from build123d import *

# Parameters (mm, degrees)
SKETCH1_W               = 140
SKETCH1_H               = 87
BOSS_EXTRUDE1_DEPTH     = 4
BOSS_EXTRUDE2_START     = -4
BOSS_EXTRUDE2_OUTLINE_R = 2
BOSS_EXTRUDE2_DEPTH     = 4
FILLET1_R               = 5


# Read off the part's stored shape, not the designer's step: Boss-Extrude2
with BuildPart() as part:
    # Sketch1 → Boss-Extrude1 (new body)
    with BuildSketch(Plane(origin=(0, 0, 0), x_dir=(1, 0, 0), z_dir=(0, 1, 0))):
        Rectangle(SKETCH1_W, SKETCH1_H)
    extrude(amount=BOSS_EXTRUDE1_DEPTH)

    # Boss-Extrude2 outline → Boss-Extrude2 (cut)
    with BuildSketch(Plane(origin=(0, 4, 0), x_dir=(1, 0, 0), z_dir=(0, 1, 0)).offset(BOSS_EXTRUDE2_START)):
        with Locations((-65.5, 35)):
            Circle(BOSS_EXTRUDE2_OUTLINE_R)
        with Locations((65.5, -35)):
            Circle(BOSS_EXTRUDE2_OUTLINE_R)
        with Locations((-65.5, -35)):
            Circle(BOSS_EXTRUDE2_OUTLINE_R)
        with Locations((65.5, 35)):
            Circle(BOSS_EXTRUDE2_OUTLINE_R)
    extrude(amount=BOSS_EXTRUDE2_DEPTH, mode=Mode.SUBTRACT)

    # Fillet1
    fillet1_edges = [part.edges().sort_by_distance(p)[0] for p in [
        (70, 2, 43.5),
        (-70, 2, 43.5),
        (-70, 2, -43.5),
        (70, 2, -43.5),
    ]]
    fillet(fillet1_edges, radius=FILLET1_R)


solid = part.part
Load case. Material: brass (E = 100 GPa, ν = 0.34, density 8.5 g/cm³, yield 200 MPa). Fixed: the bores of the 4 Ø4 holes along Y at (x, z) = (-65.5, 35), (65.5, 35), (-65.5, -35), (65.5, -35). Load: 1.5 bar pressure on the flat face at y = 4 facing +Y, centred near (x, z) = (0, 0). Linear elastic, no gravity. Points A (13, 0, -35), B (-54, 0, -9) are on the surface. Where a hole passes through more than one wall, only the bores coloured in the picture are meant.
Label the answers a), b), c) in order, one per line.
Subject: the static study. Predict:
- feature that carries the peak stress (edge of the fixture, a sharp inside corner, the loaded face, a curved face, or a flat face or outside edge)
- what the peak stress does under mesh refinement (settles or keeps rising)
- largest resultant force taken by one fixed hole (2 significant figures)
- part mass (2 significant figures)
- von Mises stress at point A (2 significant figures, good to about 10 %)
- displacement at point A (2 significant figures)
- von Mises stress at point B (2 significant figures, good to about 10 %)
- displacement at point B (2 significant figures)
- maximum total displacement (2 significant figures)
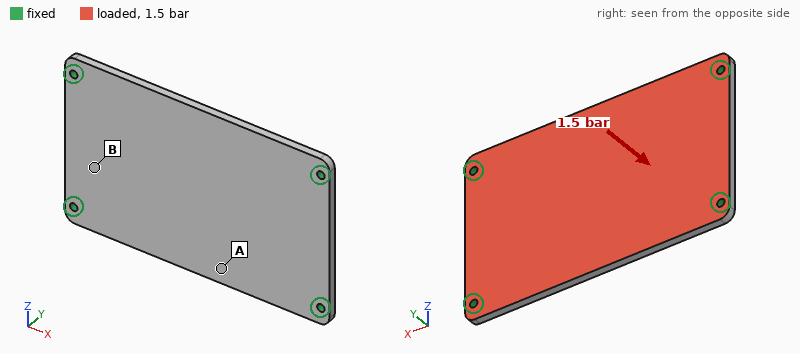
a) edge of the fixture
b) keeps rising
c) 450 N
d) 410 g
e) 46 MPa
f) 0.28 mm
g) 20 MPa
h) 0.079 mm
i) 0.31 mm
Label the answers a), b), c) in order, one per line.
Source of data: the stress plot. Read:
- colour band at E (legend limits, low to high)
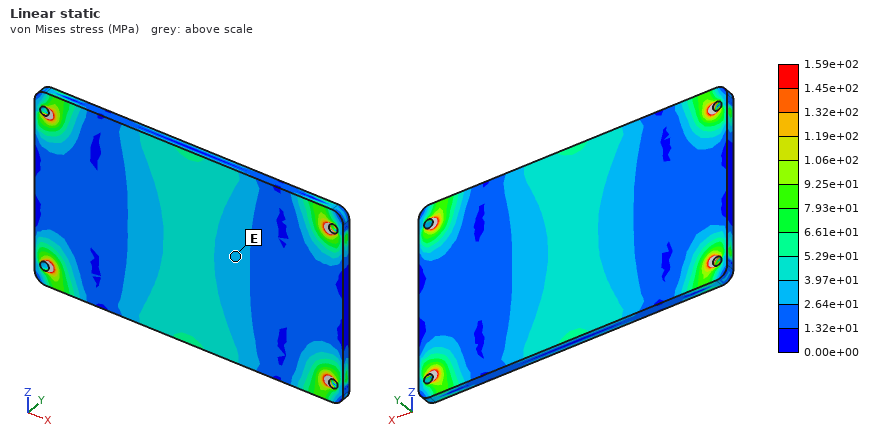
a) 2.64e+01 to 3.97e+01 MPa
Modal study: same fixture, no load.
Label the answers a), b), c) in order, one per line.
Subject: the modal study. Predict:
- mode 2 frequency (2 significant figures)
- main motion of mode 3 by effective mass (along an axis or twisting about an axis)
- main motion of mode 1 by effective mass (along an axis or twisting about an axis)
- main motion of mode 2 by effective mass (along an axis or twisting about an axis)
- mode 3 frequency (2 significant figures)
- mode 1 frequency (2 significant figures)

a) 1100 Hz
b) twisting about Z
c) along Y
d) twisting about X
e) 1900 Hz
f) 680 Hz
